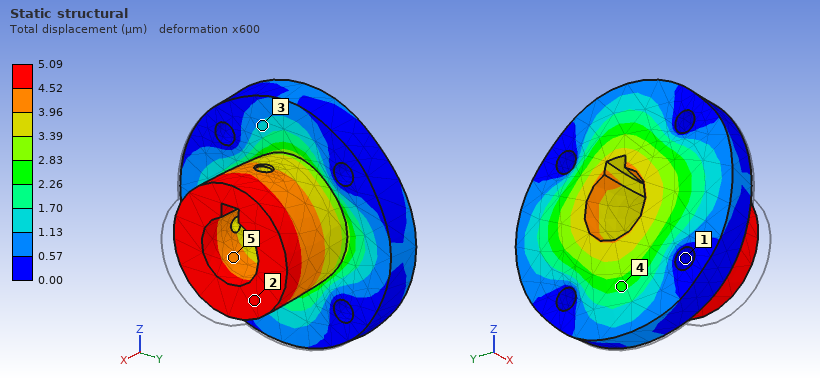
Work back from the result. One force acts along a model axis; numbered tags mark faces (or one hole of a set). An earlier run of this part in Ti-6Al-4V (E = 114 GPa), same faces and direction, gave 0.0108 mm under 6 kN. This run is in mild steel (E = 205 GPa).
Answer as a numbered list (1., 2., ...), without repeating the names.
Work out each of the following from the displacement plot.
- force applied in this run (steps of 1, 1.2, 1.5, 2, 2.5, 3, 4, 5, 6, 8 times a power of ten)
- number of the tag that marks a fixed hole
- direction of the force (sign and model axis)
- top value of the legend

1. 5 kN
2. 1
3. -X
4. 5.09 µm
